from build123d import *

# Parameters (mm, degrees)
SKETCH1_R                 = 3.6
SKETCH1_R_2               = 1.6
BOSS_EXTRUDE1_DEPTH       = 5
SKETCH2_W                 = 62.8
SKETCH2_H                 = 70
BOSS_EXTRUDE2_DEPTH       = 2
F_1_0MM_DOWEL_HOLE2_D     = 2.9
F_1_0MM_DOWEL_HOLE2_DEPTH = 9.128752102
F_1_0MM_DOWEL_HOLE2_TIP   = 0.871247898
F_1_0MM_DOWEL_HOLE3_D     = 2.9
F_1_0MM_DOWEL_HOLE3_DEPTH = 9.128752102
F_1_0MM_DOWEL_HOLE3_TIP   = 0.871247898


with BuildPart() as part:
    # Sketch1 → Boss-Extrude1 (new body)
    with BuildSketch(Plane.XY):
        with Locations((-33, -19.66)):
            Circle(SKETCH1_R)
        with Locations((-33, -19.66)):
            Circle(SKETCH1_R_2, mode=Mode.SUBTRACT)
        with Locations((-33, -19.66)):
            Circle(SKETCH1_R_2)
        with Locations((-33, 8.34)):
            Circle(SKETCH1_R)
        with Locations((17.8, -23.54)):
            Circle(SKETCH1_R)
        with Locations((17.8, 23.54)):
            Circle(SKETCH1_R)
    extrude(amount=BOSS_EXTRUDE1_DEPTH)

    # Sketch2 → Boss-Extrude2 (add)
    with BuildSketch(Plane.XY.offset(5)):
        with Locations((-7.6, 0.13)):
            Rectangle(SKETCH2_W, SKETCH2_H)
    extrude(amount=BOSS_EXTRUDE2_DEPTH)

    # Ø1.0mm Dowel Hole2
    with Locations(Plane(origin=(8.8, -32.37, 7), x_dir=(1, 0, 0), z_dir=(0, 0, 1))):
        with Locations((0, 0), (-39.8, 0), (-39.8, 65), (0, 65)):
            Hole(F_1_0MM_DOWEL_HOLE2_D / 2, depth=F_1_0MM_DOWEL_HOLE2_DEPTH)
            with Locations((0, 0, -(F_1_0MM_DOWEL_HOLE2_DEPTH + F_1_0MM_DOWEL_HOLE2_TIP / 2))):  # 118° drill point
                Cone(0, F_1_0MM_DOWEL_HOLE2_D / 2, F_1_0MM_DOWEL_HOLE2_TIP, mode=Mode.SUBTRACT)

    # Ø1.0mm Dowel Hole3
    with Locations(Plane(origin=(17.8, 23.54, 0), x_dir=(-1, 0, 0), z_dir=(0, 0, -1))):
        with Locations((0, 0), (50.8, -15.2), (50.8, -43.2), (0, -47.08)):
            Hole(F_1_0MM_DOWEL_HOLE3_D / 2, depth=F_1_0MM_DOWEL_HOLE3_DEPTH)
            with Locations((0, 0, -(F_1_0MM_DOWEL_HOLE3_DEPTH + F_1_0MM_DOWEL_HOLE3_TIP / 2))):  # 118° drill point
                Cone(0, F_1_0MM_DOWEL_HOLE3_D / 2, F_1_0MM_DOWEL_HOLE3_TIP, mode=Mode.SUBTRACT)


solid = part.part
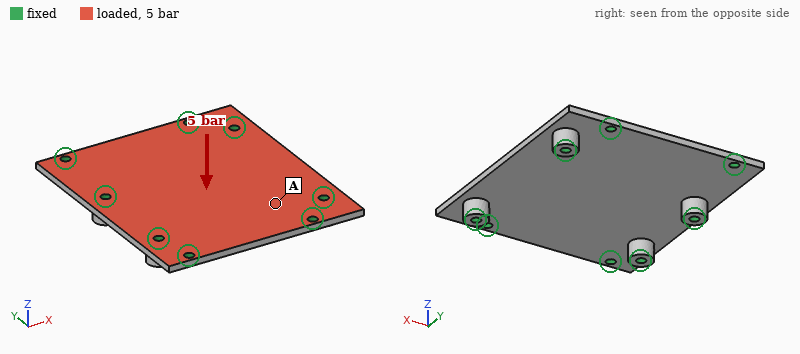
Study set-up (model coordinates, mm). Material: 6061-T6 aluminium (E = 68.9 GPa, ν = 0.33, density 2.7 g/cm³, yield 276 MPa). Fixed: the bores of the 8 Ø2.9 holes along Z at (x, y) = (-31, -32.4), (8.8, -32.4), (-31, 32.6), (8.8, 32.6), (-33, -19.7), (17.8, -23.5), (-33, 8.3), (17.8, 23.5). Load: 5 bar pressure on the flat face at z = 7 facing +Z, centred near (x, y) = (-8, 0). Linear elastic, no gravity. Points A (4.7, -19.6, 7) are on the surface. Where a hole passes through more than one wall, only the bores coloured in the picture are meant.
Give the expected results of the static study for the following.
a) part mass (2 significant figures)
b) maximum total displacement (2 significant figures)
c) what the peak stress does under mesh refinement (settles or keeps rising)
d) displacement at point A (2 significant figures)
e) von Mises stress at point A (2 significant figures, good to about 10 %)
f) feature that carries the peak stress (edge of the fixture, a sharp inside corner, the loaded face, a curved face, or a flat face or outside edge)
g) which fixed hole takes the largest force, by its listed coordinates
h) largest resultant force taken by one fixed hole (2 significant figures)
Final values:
25 g
0.23 mm
keeps rising
0.089 mm
23 MPa
edge of the fixture
(-33, 8.3)
460 N
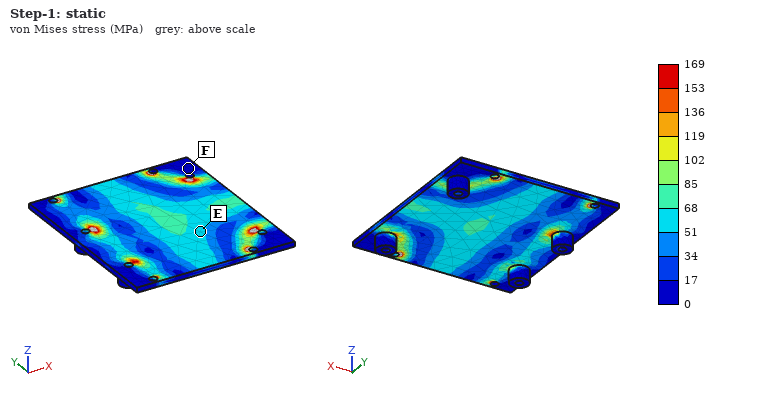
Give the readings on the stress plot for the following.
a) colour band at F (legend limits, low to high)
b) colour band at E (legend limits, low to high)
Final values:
0 to 17 MPa
51 to 68 MPa
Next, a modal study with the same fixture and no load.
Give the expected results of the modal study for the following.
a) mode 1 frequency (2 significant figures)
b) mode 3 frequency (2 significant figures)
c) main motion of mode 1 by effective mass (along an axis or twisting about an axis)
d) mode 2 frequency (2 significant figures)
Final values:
4000 Hz
6400 Hz
along Z
6300 Hz
